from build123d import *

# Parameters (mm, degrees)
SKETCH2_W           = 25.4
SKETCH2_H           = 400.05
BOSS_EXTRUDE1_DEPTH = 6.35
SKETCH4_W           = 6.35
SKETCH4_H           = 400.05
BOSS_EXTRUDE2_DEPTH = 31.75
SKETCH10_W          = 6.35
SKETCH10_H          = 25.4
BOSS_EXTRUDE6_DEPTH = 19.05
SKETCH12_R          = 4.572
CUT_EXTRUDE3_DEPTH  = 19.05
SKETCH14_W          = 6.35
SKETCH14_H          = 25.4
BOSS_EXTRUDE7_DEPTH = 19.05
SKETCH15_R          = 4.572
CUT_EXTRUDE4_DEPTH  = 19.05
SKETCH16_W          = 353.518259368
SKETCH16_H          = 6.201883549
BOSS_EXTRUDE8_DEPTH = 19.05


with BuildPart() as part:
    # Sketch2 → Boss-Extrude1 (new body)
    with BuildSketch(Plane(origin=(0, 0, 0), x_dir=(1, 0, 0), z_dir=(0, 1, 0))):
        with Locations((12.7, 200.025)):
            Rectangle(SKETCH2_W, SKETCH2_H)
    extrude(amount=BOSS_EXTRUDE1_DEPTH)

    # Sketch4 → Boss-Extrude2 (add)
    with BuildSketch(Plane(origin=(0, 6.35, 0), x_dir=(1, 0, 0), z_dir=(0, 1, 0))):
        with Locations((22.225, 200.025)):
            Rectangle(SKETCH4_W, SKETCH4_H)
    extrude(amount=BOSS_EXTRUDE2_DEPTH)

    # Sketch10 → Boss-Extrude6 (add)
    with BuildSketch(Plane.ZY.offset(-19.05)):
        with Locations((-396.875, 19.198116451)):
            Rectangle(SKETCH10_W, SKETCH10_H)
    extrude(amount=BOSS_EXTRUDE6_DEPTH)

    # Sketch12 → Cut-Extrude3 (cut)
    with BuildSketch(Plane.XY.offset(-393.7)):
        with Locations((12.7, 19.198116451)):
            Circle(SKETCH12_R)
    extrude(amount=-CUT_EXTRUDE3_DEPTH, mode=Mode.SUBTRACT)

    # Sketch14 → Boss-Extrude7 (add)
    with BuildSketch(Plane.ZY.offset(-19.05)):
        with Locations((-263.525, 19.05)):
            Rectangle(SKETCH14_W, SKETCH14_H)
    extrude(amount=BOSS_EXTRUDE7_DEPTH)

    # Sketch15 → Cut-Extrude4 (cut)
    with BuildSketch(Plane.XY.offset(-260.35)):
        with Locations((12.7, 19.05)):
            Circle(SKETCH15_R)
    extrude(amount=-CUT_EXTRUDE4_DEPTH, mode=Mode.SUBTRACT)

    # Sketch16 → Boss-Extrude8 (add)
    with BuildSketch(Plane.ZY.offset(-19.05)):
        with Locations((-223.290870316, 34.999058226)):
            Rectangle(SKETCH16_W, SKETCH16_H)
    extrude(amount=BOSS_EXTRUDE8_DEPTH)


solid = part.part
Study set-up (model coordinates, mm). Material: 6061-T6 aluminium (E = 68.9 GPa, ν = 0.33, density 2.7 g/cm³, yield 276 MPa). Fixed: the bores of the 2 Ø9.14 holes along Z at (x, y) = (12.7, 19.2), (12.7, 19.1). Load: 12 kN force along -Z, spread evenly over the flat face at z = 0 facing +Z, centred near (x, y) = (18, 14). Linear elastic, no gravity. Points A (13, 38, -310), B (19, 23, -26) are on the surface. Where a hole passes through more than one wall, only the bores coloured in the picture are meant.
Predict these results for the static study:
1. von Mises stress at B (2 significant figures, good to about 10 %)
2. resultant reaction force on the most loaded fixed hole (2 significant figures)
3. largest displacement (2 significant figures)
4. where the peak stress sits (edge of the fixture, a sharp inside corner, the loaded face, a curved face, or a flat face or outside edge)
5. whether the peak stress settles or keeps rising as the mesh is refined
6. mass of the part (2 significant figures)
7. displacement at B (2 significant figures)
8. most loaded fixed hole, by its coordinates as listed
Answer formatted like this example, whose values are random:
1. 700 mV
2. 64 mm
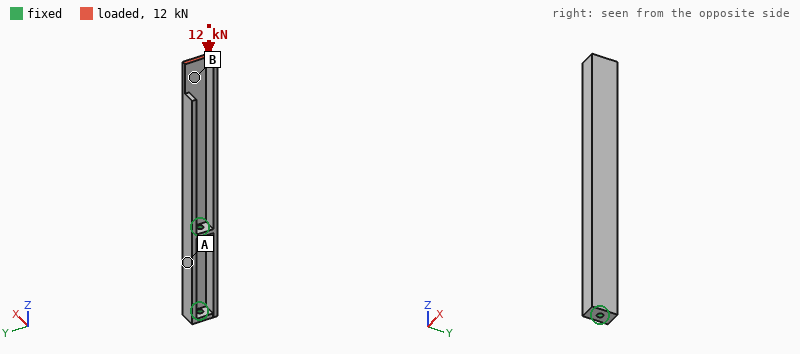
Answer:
1. 35 MPa
2. 9.2 kN
3. 0.69 mm
4. edge of the fixture
5. keeps rising
6. 520 g
7. 0.58 mm
8. (12.7, 19.1)
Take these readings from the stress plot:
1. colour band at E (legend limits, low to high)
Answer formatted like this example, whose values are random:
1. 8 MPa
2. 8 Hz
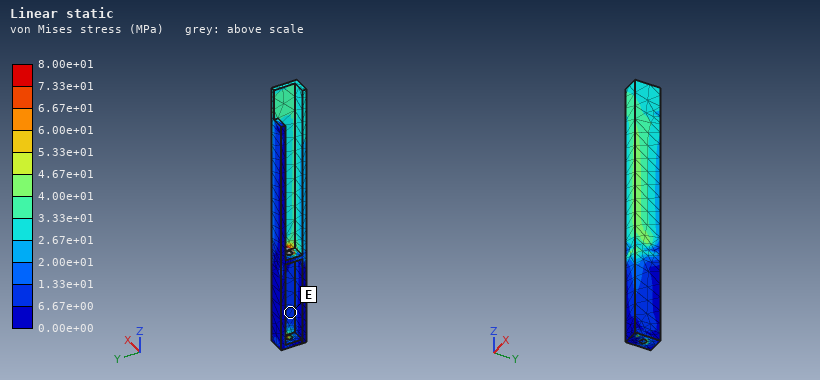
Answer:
1. 6.67e+00 to 1.33e+01 MPa
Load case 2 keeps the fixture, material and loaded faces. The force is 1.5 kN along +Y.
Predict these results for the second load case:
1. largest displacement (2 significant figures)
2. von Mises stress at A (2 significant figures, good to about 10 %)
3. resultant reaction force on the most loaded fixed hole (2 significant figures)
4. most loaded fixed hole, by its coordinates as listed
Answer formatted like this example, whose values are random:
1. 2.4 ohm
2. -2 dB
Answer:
1. 3.3 mm
2. 49 MPa
3. 4.1 kN
4. (12.7, 19.1)
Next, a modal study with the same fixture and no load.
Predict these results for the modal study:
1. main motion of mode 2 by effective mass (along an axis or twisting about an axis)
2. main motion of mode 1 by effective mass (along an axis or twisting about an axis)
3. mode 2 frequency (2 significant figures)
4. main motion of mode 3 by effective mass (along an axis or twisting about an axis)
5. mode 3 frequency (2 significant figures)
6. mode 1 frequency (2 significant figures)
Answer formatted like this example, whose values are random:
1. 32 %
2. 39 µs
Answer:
1. along Y
2. along X
3. 390 Hz
4. twisting about Z
5. 880 Hz
6. 260 Hz
